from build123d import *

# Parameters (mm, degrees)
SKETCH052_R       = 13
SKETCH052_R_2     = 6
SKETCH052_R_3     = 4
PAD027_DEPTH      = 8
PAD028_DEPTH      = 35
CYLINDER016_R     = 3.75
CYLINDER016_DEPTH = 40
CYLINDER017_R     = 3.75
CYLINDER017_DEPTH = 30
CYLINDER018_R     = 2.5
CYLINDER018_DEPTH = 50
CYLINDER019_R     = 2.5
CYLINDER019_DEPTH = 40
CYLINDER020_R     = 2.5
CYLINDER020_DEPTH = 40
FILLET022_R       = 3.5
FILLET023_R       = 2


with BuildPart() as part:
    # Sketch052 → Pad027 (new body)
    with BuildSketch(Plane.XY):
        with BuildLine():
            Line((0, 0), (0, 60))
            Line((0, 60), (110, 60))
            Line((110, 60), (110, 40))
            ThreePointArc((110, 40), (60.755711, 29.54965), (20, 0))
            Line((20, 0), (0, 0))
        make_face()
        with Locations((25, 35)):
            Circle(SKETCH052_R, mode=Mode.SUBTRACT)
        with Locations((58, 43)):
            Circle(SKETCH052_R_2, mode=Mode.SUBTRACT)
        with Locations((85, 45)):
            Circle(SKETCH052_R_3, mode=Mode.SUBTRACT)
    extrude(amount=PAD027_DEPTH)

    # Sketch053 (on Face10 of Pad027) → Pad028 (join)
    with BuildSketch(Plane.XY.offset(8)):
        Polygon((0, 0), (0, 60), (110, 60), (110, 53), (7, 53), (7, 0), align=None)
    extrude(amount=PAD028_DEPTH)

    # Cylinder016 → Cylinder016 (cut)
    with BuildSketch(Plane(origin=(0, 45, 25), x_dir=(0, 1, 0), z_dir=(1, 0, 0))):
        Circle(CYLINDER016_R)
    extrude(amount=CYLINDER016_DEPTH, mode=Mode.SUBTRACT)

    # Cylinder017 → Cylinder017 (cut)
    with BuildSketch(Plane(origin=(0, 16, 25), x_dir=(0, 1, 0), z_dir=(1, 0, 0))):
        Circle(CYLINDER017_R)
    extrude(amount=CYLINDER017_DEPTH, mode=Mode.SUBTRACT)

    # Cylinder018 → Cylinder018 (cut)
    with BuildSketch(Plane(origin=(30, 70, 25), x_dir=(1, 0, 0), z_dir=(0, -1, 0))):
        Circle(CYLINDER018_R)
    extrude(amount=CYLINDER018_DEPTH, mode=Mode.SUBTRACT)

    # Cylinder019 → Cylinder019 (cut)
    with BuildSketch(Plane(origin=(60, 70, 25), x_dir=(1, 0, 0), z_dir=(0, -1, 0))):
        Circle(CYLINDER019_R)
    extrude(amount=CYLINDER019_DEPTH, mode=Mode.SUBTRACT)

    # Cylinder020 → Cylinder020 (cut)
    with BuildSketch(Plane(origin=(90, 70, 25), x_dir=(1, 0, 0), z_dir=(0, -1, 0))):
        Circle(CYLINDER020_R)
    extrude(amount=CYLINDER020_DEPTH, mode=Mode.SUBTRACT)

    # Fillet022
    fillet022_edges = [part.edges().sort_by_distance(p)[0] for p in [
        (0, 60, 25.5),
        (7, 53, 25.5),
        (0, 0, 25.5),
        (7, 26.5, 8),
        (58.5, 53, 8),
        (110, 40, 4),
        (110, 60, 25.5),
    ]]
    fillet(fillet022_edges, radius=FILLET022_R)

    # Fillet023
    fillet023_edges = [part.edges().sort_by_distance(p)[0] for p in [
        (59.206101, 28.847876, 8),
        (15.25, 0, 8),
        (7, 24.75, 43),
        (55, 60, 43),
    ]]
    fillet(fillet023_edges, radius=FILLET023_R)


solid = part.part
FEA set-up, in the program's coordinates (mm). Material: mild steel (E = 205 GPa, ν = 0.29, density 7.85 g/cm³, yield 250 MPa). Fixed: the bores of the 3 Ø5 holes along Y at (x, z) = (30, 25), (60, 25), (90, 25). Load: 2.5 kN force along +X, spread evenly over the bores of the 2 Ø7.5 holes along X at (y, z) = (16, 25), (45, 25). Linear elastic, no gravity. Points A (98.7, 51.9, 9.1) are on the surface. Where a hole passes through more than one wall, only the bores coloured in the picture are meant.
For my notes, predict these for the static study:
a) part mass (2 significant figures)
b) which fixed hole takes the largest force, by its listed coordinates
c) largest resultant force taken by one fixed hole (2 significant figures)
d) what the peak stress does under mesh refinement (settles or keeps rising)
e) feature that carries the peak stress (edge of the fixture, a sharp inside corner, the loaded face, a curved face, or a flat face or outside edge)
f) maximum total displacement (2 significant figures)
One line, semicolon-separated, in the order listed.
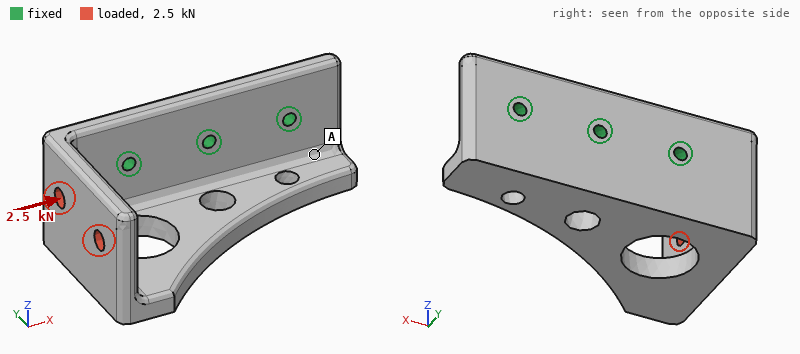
520 g; (30, 25); 1.7 kN; keeps rising; edge of the fixture; 0.10 mm
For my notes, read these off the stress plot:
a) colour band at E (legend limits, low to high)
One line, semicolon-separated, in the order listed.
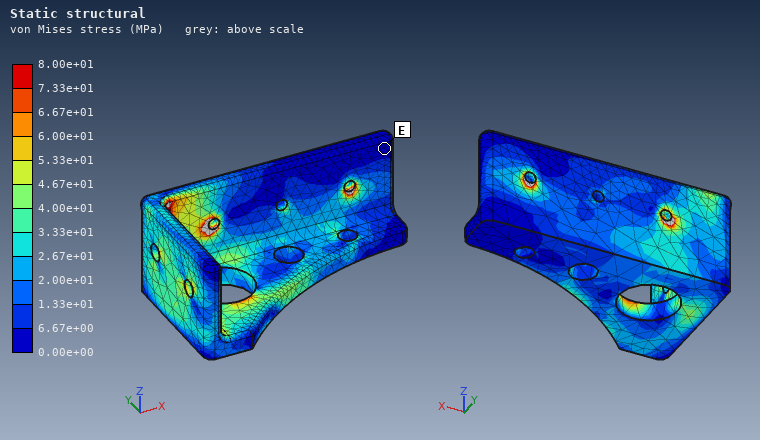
0.00e+00 to 6.67e+00 MPa
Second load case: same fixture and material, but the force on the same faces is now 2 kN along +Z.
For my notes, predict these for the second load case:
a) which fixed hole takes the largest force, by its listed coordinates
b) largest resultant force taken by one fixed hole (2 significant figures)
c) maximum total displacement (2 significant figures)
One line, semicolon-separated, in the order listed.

(30, 25); 3.1 kN; 0.15 mm
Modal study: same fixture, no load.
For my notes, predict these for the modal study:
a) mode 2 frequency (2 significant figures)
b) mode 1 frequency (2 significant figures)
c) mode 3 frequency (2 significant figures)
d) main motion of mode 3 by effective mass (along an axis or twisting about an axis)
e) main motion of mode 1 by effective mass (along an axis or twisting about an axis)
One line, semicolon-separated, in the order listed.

2500 Hz; 1400 Hz; 4000 Hz; along Y; along Z
